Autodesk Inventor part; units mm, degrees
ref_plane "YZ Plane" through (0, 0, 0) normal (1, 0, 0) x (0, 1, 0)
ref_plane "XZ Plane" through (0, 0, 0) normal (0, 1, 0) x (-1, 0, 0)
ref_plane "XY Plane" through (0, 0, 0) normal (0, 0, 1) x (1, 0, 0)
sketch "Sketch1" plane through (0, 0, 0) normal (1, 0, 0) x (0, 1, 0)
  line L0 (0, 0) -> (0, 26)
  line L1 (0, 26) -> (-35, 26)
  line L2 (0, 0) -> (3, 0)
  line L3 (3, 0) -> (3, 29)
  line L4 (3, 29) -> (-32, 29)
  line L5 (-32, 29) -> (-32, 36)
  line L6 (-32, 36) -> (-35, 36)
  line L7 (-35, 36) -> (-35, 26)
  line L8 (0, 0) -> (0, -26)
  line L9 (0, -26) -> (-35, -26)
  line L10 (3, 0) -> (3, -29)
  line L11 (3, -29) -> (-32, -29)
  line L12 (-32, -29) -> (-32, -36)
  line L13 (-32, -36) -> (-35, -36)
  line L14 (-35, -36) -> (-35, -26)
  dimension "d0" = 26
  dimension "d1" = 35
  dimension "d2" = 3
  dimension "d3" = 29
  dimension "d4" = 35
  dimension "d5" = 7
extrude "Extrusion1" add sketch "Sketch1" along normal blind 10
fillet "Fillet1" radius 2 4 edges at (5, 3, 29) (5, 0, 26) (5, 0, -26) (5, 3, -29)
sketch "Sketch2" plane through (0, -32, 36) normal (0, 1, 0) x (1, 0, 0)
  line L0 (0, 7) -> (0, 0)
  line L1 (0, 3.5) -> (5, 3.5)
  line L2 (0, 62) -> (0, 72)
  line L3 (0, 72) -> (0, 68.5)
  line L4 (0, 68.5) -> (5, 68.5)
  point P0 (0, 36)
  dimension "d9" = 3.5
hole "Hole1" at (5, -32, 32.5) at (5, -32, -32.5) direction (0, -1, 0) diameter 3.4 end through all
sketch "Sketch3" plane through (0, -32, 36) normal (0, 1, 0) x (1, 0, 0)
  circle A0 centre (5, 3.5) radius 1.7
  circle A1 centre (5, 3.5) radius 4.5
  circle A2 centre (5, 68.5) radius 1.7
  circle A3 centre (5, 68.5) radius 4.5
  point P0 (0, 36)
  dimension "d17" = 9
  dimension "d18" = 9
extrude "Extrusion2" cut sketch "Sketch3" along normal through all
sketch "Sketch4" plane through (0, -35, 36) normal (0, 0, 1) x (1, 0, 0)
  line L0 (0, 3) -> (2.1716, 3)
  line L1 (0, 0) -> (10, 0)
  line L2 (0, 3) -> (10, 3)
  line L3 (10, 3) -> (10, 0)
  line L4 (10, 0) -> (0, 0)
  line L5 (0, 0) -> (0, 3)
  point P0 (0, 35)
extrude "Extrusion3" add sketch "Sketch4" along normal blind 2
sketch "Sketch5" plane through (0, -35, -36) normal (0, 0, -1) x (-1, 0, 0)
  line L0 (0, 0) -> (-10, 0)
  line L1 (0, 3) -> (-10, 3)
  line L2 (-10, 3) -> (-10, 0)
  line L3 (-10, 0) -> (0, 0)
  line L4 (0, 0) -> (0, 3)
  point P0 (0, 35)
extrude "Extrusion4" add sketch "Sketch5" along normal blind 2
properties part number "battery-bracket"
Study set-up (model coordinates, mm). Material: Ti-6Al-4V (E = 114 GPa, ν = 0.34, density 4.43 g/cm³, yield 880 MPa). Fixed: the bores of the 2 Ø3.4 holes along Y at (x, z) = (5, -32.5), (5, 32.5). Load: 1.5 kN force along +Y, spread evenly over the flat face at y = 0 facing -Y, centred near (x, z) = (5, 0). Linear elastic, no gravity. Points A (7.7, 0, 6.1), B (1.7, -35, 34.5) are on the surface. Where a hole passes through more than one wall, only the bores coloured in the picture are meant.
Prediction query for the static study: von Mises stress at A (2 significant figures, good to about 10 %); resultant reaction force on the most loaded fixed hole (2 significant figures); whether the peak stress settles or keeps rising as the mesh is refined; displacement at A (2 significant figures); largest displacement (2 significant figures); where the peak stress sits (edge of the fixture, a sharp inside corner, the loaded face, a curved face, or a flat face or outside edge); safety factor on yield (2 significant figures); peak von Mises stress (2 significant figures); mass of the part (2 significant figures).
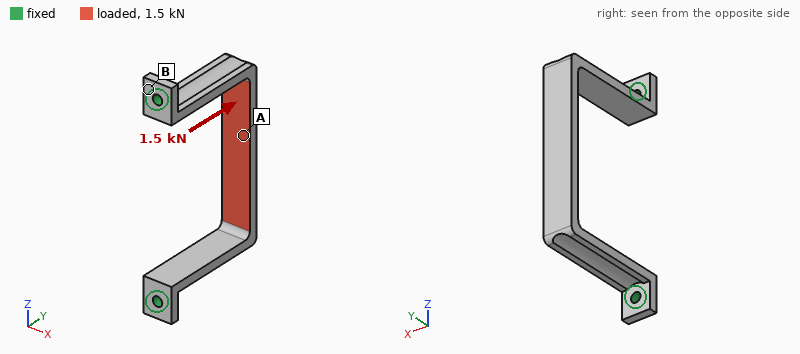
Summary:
330 MPa
790 N
settles
0.52 mm
0.57 mm
a curved face
1.7
510 MPa
18 g
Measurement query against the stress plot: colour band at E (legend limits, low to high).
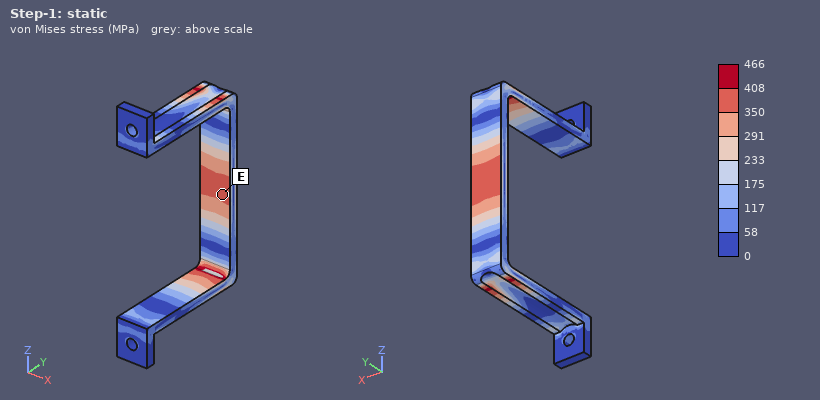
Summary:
350 to 408 MPa
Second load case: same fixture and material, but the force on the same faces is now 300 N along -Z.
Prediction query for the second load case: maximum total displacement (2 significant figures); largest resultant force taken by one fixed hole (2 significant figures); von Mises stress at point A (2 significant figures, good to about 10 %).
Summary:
0.44 mm
170 N
40 MPa
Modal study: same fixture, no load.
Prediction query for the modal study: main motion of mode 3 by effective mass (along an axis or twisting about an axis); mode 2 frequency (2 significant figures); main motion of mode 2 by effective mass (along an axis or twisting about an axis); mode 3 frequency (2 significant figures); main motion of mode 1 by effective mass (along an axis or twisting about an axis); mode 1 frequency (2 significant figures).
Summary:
twisting about Y
1800 Hz
along X
2800 Hz
along Z
1300 Hz
